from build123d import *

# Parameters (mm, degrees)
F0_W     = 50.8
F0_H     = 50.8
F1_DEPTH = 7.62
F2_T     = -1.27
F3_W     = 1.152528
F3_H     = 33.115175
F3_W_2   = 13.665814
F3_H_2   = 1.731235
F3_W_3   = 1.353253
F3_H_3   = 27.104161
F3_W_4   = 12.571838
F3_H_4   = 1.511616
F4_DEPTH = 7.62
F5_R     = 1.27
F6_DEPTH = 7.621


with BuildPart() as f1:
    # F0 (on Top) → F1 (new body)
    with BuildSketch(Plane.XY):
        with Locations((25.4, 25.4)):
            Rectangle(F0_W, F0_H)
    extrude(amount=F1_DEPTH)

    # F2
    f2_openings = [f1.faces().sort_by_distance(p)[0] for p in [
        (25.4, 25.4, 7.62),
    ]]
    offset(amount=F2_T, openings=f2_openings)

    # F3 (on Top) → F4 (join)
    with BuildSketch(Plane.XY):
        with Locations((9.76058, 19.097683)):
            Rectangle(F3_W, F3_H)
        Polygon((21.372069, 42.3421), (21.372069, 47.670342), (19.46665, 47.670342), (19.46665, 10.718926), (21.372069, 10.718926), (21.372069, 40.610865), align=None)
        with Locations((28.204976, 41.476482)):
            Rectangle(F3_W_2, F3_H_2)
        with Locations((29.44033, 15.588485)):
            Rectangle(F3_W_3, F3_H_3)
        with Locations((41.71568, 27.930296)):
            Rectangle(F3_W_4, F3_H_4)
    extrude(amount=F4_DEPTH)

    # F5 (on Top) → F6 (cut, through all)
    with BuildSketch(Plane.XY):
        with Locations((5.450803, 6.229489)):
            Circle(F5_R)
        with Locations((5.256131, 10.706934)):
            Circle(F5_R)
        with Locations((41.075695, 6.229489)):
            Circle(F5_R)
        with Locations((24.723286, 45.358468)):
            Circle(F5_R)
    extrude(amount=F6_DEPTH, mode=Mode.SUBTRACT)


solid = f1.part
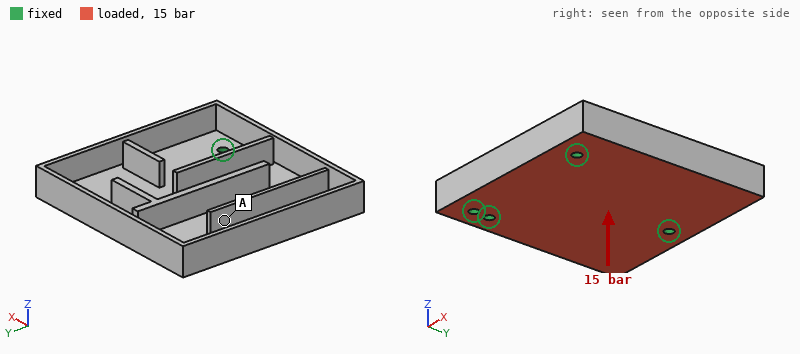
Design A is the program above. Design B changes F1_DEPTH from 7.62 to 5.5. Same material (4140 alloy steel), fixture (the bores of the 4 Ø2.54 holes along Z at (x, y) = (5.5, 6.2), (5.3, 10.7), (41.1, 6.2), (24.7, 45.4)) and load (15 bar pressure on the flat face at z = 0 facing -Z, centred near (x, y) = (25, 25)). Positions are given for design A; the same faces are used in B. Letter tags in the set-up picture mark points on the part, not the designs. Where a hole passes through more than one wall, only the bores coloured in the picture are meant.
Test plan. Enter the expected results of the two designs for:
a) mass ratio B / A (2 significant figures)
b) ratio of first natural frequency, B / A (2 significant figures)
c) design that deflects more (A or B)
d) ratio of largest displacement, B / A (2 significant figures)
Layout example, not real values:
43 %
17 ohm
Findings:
0.91
1.0
B
1.4
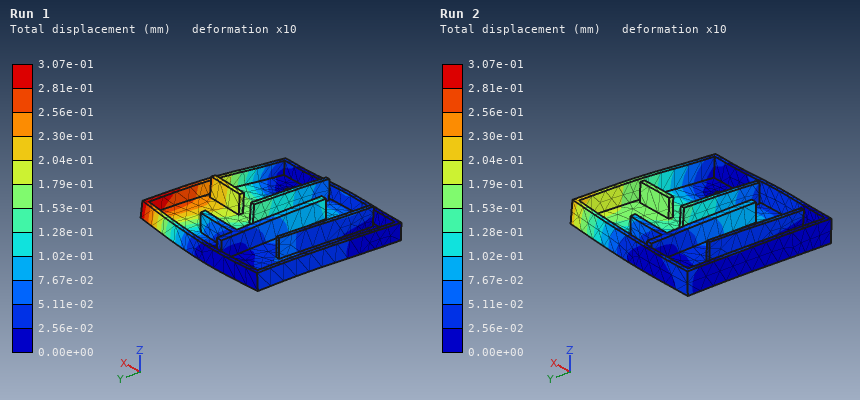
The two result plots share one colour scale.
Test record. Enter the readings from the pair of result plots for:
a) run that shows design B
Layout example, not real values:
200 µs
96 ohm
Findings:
Run 1
